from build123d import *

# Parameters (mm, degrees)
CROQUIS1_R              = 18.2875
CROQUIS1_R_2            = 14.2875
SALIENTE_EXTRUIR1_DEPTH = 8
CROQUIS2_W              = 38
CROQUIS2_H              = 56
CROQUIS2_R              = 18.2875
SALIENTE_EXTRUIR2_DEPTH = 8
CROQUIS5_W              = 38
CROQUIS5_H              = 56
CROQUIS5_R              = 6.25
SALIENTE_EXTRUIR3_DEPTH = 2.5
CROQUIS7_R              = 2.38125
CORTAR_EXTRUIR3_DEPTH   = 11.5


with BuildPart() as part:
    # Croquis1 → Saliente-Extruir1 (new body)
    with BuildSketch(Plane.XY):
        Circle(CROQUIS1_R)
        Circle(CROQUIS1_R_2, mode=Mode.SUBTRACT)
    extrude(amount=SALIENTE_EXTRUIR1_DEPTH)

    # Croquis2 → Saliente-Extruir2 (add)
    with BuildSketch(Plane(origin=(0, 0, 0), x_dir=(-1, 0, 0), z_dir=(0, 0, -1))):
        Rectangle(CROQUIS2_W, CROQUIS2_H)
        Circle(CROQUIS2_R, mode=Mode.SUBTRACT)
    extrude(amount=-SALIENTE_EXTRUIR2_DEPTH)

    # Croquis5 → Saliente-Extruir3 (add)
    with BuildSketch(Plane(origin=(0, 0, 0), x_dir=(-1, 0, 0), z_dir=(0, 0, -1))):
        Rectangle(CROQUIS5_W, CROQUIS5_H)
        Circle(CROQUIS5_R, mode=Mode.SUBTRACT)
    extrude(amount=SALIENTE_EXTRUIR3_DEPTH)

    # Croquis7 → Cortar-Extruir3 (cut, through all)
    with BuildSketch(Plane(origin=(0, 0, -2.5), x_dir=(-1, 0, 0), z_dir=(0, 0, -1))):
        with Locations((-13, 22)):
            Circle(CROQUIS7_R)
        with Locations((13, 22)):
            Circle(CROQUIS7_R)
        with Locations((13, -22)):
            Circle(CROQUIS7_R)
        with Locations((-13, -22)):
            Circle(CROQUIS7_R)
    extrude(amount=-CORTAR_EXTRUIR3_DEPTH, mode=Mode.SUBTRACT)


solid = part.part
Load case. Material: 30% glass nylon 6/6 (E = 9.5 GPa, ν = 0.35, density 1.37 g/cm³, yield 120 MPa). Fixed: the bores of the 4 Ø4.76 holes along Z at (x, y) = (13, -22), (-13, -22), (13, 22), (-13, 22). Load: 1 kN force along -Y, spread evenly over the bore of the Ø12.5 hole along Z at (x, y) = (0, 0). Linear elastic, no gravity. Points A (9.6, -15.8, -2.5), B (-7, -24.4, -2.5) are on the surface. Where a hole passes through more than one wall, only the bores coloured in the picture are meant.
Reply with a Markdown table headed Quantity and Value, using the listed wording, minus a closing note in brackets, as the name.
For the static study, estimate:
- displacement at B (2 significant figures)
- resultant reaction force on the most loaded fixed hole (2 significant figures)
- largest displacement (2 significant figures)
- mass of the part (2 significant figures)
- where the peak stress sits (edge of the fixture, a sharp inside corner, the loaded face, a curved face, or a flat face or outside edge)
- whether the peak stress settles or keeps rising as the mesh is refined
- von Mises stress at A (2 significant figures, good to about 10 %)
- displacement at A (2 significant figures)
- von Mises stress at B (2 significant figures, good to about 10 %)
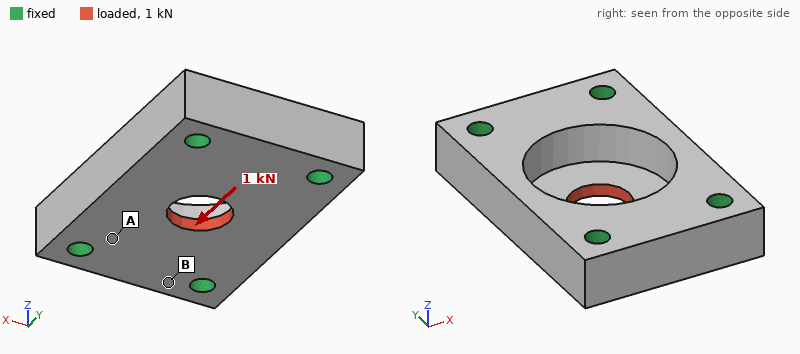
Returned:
| Quantity | Value |
|---|---|
| displacement at B | 2.5 µm |
| resultant reaction force on the most loaded fixed hole | 260 N |
| largest displacement | 16 µm |
| mass of the part | 22 g |
| where the peak stress sits | a sharp inside corner |
| whether the peak stress settles or keeps rising as the mesh is refined | keeps rising |
| von Mises stress at A | 6.0 MPa |
| displacement at A | 3.4 µm |
| von Mises stress at B | 2.5 MPa |
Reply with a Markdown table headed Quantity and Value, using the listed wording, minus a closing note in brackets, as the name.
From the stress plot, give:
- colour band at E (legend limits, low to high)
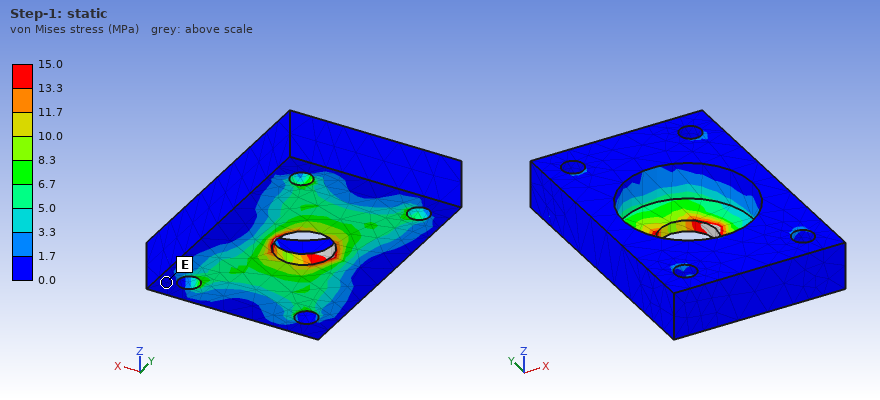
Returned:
| Quantity | Value |
|---|---|
| colour band at E | 0.0 to 1.7 MPa |
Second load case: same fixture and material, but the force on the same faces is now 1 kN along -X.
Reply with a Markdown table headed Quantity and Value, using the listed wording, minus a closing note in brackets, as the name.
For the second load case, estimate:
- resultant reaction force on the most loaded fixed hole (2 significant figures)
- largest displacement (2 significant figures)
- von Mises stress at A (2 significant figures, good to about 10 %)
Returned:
| Quantity | Value |
|---|---|
| resultant reaction force on the most loaded fixed hole | 300 N |
| largest displacement | 26 µm |
| von Mises stress at A | 5.9 MPa |
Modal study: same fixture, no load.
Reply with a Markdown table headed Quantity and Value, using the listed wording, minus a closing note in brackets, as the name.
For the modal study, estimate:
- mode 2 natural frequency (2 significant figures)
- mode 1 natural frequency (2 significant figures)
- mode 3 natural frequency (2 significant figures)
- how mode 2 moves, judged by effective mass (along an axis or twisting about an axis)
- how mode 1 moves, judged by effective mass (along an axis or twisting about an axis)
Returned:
| Quantity | Value |
|---|---|
| mode 2 natural frequency | 14 kHz |
| mode 1 natural frequency | 12 kHz |
| mode 3 natural frequency | 16 kHz |
| how mode 2 moves, judged by effective mass | twisting about Y |
| how mode 1 moves, judged by effective mass | along Z |
